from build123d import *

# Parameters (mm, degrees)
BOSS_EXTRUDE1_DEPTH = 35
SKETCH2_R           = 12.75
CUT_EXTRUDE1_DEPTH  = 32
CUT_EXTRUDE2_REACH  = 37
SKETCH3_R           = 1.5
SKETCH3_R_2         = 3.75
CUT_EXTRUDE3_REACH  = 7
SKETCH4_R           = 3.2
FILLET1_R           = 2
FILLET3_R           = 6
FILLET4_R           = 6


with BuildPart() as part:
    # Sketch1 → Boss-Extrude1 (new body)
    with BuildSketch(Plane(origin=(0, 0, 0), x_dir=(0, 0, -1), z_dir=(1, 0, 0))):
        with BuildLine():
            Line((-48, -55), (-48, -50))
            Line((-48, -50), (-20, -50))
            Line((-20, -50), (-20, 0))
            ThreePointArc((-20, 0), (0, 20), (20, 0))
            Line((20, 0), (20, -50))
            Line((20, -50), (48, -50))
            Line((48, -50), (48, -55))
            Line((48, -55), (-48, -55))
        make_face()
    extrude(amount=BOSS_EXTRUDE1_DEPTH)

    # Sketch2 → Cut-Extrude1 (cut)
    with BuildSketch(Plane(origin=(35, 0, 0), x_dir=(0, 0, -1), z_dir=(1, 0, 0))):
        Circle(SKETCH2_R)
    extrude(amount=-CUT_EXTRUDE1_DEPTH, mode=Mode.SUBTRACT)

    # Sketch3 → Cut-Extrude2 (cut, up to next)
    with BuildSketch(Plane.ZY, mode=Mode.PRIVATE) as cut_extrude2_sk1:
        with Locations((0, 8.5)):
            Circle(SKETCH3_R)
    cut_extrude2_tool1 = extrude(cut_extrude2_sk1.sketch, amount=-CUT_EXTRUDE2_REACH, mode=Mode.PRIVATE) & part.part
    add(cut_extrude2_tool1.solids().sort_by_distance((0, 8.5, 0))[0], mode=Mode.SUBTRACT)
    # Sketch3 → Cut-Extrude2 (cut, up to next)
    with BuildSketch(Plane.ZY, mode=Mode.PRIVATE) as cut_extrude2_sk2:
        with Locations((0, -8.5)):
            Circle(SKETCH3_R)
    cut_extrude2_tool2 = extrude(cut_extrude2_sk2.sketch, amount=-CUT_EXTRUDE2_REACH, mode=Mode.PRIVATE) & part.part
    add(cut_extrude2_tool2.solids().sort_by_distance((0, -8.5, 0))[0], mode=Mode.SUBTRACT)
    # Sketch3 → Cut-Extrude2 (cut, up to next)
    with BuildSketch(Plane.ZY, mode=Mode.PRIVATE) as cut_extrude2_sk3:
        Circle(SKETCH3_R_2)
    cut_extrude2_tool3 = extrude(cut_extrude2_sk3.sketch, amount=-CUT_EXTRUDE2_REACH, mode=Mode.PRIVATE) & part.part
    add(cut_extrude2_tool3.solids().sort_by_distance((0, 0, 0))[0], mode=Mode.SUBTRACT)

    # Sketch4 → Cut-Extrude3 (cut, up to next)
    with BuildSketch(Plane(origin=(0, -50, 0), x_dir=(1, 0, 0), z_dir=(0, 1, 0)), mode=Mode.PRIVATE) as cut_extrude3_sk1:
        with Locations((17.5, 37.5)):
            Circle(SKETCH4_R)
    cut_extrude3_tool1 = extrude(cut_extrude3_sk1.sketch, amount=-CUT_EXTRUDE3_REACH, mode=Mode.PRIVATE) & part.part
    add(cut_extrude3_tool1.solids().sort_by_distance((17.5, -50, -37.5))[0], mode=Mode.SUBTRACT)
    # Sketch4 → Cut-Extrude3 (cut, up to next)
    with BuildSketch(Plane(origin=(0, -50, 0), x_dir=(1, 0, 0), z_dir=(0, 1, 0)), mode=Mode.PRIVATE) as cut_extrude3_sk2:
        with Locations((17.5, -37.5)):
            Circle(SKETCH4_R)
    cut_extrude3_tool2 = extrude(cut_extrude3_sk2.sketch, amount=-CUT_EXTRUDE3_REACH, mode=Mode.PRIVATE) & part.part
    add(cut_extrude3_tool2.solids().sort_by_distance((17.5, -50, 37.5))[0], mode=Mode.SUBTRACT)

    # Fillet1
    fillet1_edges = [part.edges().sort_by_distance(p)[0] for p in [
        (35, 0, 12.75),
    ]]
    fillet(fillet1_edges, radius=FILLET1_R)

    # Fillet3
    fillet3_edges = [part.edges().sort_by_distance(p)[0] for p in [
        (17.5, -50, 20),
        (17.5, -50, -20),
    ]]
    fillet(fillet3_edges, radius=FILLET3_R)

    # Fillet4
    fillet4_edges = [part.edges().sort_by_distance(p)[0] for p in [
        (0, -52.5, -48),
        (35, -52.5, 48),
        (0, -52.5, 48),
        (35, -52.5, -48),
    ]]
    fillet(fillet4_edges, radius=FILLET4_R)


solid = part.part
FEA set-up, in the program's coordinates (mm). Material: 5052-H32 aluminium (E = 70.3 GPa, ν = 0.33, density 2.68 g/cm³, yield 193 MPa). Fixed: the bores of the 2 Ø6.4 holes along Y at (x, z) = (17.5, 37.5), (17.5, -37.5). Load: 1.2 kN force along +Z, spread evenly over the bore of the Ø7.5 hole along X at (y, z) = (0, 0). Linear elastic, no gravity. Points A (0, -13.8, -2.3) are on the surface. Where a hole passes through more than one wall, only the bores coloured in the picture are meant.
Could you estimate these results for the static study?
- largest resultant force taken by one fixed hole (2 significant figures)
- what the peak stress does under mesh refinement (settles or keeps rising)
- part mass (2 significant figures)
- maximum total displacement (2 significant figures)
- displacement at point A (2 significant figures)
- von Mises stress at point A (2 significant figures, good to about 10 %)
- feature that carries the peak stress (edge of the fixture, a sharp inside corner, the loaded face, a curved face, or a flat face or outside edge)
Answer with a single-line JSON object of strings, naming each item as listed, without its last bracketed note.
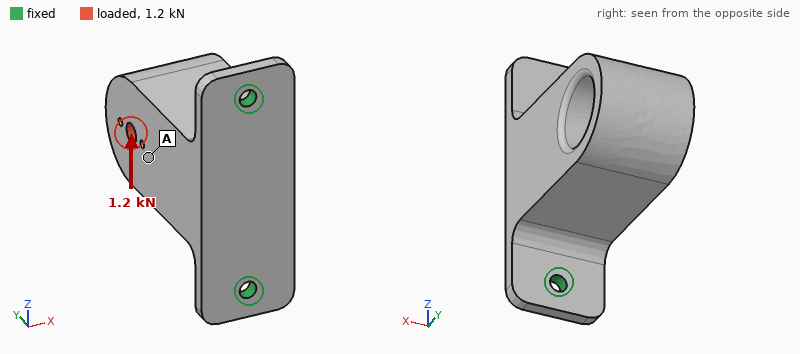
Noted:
{"largest resultant force taken by one fixed hole": "1.2 kN", "what the peak stress does under mesh refinement": "keeps rising", "part mass": "250 g", "maximum total displacement": "73 µm", "displacement at point A": "38 µm", "von Mises stress at point A": "8.7 MPa", "feature that carries the peak stress": "edge of the fixture"}
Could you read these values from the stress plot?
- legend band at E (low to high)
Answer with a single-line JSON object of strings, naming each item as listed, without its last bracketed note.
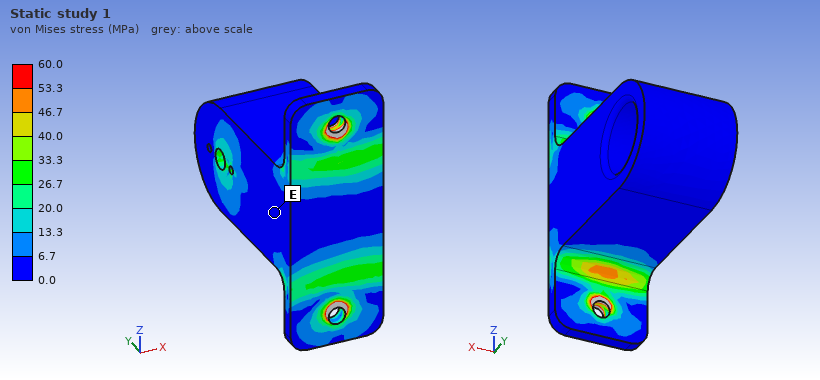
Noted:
{"legend band at E": "0.0 to 6.7 MPa"}
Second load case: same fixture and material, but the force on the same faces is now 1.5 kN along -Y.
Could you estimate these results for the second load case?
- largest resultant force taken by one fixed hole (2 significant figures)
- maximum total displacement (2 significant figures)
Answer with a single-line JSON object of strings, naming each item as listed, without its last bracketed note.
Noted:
{"largest resultant force taken by one fixed hole": "890 N", "maximum total displacement": "0.29 mm"}
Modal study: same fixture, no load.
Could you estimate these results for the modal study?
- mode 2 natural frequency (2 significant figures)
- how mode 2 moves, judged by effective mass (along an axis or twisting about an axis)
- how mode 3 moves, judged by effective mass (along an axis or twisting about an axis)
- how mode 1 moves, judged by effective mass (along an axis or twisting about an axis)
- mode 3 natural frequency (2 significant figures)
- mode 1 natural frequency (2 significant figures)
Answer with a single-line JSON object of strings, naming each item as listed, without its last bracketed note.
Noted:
{"mode 2 natural frequency": "2300 Hz", "how mode 2 moves, judged by effective mass": "along Z", "how mode 3 moves, judged by effective mass": "along Y", "how mode 1 moves, judged by effective mass": "along X", "mode 3 natural frequency": "3000 Hz", "mode 1 natural frequency": "720 Hz"}
